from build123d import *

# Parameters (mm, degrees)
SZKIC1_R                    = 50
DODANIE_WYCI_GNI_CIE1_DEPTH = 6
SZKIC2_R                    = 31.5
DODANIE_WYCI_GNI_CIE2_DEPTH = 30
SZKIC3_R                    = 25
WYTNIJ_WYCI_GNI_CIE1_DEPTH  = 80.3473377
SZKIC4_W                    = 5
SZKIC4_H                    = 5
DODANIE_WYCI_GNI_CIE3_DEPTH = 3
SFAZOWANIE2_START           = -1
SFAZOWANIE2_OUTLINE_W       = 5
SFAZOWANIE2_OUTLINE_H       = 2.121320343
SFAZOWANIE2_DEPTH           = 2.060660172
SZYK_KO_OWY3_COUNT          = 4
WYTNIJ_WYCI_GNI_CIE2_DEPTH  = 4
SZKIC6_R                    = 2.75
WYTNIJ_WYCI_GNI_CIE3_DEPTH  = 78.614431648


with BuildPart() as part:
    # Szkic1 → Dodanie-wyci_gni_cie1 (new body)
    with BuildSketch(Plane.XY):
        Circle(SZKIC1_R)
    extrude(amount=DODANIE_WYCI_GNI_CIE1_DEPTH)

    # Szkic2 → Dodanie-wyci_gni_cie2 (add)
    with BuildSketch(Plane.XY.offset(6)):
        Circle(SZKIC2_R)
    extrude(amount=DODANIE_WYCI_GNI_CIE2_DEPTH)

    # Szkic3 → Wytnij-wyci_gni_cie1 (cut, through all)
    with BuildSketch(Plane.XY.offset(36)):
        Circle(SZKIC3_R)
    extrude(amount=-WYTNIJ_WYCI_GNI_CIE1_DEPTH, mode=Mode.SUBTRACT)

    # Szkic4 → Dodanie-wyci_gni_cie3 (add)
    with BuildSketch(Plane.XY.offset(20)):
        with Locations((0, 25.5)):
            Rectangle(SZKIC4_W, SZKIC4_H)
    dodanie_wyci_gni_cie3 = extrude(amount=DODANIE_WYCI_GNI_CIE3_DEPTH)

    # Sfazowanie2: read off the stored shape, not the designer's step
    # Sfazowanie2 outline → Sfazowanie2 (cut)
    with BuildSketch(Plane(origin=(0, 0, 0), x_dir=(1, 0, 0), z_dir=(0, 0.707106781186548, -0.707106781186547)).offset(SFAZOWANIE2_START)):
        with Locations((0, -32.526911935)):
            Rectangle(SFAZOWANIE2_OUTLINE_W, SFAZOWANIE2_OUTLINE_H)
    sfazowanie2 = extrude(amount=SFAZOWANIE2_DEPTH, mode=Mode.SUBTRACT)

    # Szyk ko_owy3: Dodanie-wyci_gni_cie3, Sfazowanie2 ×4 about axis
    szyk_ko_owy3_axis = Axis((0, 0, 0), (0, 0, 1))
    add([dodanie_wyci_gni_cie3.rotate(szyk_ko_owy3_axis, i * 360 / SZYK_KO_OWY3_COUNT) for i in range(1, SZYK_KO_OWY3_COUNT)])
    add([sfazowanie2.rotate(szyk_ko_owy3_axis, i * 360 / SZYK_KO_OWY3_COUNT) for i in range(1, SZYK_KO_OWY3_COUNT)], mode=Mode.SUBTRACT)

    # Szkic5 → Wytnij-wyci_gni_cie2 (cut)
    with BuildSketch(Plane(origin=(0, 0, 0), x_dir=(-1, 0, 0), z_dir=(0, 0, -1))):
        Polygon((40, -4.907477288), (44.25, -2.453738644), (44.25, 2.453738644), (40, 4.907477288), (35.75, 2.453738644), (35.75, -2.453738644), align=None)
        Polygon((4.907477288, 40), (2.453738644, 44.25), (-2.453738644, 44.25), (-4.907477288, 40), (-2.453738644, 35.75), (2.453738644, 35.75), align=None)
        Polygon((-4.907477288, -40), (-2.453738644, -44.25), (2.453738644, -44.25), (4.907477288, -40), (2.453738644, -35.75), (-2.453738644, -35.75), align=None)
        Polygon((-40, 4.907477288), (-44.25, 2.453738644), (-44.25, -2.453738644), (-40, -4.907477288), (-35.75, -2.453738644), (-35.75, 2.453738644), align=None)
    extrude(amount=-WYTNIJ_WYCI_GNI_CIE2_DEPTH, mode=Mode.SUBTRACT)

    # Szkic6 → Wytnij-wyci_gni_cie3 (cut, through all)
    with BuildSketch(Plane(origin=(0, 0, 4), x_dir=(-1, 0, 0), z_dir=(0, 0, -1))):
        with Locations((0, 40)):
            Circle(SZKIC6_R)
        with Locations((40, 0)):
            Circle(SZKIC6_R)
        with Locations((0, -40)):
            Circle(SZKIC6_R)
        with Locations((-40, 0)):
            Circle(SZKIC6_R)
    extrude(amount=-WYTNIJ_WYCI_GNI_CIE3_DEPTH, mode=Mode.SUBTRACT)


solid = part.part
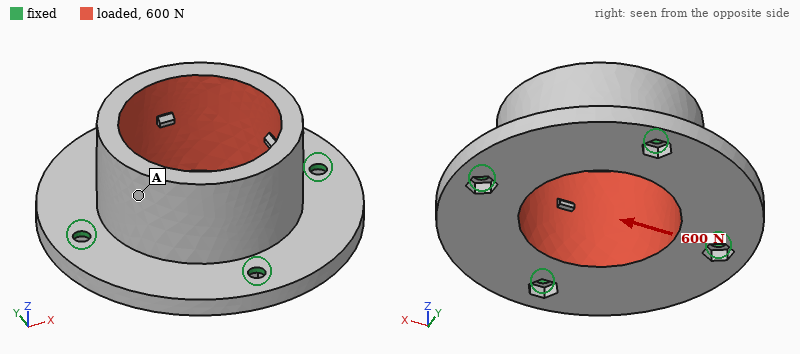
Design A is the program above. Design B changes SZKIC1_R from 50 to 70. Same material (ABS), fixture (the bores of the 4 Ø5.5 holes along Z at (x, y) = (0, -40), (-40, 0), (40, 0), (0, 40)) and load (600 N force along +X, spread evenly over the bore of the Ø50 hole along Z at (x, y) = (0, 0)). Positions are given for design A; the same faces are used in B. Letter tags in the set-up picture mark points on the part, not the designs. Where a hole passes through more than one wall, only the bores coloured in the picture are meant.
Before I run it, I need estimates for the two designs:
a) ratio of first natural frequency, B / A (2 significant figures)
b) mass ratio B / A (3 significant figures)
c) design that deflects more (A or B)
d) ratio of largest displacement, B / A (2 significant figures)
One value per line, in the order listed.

0.45
1.66
A
0.91
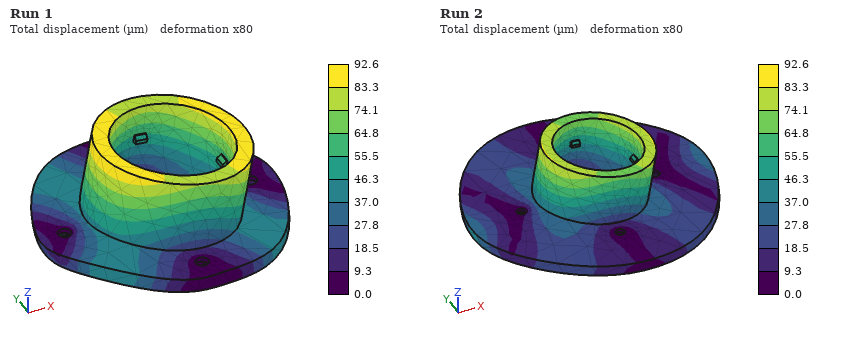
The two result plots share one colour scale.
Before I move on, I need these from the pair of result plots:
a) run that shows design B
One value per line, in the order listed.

Run 2
